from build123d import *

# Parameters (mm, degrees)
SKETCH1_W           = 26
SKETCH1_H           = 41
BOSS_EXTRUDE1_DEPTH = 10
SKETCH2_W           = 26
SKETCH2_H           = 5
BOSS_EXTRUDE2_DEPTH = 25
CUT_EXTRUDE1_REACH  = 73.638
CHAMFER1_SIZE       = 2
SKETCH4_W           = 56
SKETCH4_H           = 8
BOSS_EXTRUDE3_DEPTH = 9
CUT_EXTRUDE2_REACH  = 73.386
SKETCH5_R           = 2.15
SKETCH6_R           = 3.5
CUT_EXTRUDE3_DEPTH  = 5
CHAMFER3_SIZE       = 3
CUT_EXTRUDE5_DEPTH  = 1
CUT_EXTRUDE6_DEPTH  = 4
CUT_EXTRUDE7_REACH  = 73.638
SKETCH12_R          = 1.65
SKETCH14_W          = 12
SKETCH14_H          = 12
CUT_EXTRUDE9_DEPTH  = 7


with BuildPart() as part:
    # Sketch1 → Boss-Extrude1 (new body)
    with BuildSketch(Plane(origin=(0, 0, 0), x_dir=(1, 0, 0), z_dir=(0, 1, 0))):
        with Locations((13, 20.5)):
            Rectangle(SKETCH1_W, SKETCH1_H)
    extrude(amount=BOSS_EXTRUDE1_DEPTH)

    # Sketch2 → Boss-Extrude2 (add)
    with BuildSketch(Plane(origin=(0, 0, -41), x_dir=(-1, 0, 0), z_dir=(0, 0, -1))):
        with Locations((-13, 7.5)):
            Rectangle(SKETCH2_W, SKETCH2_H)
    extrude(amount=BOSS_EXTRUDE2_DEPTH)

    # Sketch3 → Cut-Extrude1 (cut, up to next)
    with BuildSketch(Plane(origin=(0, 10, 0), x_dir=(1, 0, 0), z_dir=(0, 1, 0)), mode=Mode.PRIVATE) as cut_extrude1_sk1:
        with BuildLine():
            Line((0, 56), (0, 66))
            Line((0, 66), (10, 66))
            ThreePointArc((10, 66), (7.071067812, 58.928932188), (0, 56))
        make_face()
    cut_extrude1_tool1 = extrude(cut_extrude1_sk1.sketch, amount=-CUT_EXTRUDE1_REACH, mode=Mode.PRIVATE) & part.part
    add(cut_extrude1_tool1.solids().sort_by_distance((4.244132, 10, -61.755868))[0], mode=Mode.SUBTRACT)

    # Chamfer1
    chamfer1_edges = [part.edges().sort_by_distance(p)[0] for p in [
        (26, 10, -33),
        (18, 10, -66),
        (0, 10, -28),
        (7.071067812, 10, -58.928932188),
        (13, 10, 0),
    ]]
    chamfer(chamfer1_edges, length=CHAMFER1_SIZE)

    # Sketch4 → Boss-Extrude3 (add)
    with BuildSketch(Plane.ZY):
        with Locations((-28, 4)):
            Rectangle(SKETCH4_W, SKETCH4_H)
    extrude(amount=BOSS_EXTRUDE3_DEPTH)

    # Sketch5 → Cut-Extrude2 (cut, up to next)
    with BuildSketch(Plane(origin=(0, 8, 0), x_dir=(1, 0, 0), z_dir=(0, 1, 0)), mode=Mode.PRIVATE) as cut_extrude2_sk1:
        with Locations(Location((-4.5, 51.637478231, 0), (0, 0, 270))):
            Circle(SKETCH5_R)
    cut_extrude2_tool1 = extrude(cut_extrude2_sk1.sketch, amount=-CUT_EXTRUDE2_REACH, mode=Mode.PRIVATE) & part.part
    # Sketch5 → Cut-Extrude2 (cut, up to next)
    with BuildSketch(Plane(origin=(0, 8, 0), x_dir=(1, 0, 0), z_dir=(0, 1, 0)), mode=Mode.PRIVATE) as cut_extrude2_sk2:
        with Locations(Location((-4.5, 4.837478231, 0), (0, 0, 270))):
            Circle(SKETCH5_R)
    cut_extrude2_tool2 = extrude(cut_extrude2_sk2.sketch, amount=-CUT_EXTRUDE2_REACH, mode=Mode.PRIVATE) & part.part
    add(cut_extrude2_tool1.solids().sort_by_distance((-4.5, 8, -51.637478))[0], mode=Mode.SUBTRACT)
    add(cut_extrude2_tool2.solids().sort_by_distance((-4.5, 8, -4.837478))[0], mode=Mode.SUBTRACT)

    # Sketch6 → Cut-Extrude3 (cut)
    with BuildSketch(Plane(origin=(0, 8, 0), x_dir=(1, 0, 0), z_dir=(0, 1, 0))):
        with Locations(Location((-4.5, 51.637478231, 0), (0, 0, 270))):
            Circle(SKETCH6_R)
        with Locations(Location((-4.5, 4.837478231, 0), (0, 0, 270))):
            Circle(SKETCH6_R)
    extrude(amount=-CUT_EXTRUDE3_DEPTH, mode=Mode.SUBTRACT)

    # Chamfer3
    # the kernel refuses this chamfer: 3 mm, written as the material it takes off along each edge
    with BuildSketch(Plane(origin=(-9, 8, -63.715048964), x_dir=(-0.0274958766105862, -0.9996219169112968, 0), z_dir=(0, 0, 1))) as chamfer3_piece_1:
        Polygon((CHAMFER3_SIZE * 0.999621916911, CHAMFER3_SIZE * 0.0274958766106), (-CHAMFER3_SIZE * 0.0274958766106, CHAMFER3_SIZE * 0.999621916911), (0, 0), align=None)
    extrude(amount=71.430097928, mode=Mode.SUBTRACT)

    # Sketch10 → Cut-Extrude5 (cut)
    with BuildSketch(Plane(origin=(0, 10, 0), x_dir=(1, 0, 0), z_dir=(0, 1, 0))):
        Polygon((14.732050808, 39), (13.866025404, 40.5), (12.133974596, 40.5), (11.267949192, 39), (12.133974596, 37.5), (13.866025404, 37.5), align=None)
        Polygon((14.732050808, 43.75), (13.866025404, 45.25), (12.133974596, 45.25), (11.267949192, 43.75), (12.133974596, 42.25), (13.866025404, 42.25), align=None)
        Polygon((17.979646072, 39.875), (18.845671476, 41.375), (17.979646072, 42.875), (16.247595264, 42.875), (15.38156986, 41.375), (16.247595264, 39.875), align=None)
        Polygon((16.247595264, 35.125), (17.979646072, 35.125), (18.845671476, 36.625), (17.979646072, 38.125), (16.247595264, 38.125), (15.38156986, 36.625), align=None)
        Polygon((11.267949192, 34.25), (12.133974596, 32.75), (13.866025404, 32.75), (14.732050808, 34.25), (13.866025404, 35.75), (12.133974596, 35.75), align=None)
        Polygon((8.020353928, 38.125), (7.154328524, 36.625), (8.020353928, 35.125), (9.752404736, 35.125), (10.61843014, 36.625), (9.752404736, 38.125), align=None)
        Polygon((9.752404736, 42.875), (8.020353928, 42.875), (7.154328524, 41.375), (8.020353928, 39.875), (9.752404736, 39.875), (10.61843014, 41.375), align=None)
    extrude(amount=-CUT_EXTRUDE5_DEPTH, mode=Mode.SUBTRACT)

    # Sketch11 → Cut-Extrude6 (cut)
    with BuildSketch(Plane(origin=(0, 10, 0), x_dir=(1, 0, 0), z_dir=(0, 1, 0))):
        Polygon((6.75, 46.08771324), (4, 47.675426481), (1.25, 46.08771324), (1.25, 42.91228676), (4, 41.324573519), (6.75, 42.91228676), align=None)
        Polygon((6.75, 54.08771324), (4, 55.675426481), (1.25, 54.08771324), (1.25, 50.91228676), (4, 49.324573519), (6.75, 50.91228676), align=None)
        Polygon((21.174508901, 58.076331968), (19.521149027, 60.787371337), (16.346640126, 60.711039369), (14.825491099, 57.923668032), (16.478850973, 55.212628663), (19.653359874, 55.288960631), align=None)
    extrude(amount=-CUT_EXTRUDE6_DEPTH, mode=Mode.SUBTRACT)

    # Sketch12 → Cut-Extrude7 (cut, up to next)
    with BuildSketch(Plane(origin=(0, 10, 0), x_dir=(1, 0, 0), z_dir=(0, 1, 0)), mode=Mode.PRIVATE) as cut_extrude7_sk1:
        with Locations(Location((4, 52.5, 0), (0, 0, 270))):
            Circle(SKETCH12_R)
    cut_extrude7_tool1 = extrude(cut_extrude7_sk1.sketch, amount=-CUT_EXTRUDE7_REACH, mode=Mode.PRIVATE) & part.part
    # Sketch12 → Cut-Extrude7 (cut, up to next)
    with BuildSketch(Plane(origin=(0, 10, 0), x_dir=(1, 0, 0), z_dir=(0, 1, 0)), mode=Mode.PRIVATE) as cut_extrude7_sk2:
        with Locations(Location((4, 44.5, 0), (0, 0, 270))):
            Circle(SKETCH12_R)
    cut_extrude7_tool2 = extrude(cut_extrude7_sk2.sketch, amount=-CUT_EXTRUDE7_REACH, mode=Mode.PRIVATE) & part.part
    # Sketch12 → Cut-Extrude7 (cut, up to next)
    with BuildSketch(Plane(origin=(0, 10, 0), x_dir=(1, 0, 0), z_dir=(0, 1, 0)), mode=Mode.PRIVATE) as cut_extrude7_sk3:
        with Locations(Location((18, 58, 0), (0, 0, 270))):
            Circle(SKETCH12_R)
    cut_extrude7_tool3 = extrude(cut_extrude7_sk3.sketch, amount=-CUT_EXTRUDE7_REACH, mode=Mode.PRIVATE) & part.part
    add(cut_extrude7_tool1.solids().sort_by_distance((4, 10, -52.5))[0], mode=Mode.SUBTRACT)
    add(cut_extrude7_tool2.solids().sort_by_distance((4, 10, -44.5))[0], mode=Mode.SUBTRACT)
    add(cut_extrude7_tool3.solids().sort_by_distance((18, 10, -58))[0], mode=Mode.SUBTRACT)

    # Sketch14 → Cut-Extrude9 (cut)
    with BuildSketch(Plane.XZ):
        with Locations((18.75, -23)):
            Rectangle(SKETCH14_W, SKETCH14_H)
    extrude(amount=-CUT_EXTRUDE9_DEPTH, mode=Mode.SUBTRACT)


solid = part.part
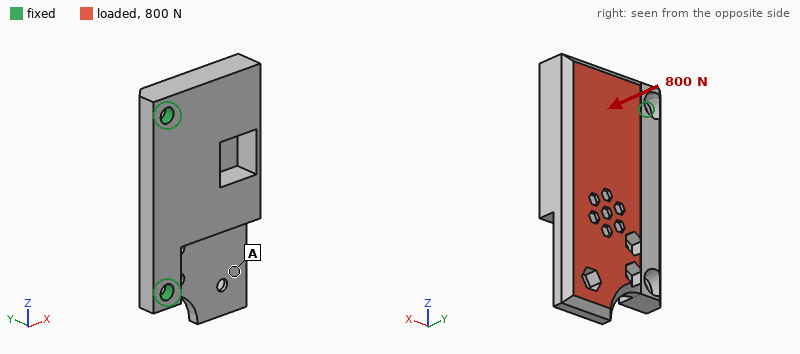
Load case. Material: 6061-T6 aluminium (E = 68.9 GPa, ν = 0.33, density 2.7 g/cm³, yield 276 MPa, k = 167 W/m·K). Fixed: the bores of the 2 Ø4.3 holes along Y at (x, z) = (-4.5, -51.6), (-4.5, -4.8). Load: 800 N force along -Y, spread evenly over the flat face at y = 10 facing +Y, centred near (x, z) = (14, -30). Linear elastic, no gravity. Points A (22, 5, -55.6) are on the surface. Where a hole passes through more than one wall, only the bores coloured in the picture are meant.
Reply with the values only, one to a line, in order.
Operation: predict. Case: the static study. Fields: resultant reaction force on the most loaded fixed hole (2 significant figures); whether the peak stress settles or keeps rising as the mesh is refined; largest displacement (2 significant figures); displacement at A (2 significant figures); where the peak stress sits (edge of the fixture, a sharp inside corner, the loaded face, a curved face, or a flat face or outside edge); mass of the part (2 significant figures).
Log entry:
470 N
keeps rising
0.20 mm
0.16 mm
edge of the fixture
41 g
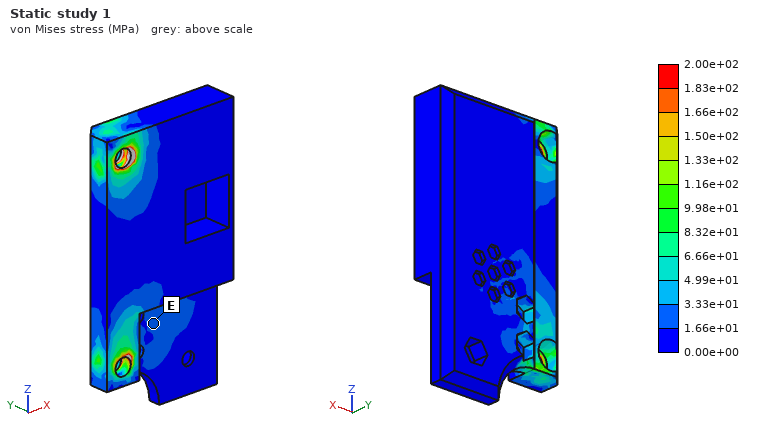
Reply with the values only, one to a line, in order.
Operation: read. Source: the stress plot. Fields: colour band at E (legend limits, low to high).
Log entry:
1.66e+01 to 3.33e+01 MPa
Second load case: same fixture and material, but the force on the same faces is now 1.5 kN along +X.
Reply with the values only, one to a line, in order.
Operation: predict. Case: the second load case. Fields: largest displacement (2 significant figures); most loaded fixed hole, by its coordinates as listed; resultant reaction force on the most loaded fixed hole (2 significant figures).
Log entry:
0.15 mm
(-4.5, -51.6)
820 N
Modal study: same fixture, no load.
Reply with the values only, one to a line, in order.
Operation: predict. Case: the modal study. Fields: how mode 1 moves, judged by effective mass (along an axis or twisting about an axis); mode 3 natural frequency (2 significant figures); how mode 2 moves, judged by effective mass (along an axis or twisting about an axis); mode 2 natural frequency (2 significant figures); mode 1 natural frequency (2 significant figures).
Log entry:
along Y
9500 Hz
twisting about X
5700 Hz
2400 Hz
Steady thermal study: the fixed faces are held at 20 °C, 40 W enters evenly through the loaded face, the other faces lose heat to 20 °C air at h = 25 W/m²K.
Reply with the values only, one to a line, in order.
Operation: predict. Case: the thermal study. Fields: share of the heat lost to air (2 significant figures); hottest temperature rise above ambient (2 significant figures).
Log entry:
5.7 %
27 K
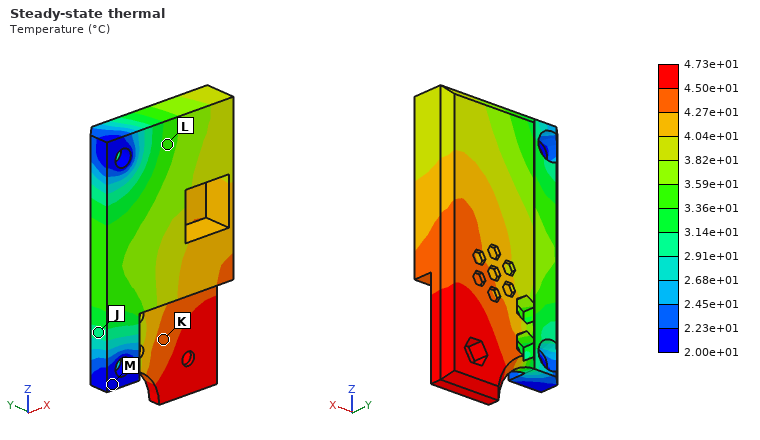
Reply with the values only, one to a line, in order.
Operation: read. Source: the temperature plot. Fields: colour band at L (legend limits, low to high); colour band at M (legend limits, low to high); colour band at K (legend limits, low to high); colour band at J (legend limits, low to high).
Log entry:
3.36e+01 to 3.59e+01 °C
2.00e+01 to 2.23e+01 °C
4.27e+01 to 4.50e+01 °C
2.91e+01 to 3.14e+01 °C
